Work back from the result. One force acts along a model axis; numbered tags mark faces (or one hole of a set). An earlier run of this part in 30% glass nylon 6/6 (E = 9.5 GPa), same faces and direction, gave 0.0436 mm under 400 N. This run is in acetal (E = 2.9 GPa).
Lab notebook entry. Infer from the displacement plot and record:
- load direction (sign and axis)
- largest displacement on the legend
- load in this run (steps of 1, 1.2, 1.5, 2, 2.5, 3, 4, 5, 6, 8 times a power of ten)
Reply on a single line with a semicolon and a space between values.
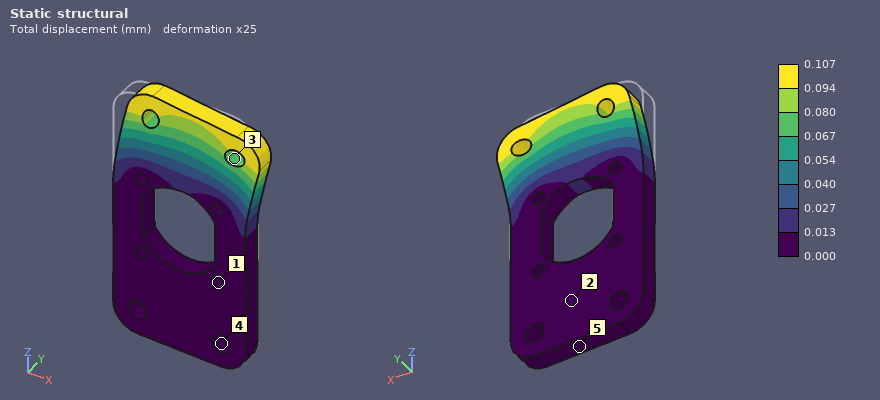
+X; 0.107 mm; 300 N
